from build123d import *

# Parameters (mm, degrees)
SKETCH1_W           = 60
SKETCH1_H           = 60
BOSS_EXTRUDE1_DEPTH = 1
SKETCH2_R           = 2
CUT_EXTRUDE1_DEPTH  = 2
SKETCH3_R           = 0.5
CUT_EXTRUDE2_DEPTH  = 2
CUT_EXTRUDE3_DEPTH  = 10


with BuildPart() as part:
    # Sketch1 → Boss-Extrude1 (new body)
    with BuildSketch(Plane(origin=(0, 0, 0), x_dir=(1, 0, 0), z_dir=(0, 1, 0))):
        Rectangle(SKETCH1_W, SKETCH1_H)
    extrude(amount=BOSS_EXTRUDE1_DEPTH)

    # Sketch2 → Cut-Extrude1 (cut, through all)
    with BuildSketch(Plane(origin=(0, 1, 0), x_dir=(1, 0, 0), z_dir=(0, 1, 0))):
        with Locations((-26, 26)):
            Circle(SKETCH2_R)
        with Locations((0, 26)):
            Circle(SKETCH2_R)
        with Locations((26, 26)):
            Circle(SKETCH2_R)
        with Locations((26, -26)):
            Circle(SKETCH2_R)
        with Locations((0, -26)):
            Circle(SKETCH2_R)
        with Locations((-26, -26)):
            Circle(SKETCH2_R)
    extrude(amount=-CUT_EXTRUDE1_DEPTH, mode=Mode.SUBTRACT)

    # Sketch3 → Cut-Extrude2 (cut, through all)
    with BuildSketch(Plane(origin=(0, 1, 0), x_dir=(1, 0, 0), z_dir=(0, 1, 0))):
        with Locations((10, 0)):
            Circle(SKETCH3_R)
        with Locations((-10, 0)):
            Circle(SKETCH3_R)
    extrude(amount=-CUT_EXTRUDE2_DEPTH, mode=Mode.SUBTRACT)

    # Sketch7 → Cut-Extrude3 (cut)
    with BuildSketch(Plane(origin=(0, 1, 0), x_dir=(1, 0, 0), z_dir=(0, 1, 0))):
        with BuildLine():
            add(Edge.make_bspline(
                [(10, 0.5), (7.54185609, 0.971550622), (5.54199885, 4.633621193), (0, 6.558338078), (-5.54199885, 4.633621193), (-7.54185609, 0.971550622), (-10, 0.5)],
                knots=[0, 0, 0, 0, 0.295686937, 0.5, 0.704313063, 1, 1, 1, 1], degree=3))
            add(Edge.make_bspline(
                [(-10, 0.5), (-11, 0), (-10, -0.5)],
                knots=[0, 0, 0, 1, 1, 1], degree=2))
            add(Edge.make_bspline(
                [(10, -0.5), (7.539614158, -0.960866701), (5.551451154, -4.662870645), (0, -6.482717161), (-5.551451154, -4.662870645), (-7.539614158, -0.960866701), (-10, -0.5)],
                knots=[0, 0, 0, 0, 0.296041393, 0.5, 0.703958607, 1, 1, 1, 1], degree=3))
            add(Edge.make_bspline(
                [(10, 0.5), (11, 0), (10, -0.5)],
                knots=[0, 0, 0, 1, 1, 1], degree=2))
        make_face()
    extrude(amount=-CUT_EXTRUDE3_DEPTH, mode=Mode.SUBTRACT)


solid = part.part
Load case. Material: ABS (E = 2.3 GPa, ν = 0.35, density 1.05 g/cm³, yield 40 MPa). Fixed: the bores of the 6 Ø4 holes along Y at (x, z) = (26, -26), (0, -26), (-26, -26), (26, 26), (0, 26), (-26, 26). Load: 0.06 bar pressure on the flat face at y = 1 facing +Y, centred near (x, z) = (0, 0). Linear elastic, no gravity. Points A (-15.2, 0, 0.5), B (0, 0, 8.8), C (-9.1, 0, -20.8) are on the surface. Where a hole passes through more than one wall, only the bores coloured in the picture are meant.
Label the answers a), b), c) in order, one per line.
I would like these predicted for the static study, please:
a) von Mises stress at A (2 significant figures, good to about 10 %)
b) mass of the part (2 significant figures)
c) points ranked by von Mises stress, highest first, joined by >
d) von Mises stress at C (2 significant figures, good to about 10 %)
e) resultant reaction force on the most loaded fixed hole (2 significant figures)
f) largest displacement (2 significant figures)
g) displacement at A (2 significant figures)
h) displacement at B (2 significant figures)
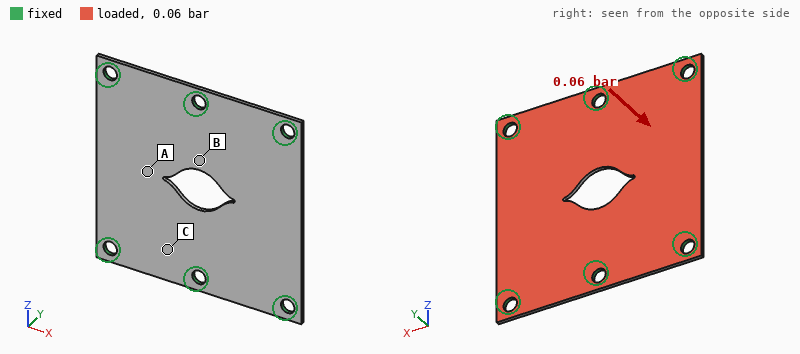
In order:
a) 4.4 MPa
b) 3.5 g
c) A > C > B
d) 2.7 MPa
e) 4.4 N
f) 0.65 mm
g) 0.59 mm
h) 0.48 mm
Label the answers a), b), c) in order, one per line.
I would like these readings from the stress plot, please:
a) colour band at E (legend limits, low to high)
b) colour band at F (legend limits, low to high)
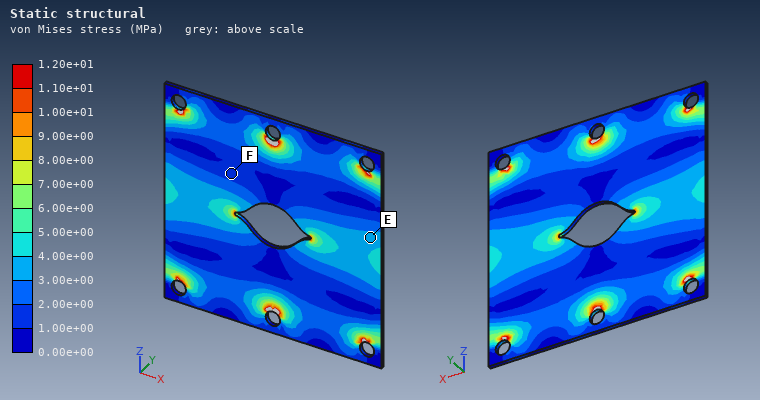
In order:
a) 3.00e+00 to 4.00e+00 MPa
b) 1.00e+00 to 2.00e+00 MPa
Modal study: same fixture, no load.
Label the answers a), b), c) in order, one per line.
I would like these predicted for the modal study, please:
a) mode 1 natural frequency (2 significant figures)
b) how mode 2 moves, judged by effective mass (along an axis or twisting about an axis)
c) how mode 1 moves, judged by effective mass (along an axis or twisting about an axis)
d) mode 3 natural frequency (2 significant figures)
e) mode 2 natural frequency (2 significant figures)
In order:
a) 580 Hz
b) twisting about Z
c) along Y
d) 1000 Hz
e) 680 Hz
